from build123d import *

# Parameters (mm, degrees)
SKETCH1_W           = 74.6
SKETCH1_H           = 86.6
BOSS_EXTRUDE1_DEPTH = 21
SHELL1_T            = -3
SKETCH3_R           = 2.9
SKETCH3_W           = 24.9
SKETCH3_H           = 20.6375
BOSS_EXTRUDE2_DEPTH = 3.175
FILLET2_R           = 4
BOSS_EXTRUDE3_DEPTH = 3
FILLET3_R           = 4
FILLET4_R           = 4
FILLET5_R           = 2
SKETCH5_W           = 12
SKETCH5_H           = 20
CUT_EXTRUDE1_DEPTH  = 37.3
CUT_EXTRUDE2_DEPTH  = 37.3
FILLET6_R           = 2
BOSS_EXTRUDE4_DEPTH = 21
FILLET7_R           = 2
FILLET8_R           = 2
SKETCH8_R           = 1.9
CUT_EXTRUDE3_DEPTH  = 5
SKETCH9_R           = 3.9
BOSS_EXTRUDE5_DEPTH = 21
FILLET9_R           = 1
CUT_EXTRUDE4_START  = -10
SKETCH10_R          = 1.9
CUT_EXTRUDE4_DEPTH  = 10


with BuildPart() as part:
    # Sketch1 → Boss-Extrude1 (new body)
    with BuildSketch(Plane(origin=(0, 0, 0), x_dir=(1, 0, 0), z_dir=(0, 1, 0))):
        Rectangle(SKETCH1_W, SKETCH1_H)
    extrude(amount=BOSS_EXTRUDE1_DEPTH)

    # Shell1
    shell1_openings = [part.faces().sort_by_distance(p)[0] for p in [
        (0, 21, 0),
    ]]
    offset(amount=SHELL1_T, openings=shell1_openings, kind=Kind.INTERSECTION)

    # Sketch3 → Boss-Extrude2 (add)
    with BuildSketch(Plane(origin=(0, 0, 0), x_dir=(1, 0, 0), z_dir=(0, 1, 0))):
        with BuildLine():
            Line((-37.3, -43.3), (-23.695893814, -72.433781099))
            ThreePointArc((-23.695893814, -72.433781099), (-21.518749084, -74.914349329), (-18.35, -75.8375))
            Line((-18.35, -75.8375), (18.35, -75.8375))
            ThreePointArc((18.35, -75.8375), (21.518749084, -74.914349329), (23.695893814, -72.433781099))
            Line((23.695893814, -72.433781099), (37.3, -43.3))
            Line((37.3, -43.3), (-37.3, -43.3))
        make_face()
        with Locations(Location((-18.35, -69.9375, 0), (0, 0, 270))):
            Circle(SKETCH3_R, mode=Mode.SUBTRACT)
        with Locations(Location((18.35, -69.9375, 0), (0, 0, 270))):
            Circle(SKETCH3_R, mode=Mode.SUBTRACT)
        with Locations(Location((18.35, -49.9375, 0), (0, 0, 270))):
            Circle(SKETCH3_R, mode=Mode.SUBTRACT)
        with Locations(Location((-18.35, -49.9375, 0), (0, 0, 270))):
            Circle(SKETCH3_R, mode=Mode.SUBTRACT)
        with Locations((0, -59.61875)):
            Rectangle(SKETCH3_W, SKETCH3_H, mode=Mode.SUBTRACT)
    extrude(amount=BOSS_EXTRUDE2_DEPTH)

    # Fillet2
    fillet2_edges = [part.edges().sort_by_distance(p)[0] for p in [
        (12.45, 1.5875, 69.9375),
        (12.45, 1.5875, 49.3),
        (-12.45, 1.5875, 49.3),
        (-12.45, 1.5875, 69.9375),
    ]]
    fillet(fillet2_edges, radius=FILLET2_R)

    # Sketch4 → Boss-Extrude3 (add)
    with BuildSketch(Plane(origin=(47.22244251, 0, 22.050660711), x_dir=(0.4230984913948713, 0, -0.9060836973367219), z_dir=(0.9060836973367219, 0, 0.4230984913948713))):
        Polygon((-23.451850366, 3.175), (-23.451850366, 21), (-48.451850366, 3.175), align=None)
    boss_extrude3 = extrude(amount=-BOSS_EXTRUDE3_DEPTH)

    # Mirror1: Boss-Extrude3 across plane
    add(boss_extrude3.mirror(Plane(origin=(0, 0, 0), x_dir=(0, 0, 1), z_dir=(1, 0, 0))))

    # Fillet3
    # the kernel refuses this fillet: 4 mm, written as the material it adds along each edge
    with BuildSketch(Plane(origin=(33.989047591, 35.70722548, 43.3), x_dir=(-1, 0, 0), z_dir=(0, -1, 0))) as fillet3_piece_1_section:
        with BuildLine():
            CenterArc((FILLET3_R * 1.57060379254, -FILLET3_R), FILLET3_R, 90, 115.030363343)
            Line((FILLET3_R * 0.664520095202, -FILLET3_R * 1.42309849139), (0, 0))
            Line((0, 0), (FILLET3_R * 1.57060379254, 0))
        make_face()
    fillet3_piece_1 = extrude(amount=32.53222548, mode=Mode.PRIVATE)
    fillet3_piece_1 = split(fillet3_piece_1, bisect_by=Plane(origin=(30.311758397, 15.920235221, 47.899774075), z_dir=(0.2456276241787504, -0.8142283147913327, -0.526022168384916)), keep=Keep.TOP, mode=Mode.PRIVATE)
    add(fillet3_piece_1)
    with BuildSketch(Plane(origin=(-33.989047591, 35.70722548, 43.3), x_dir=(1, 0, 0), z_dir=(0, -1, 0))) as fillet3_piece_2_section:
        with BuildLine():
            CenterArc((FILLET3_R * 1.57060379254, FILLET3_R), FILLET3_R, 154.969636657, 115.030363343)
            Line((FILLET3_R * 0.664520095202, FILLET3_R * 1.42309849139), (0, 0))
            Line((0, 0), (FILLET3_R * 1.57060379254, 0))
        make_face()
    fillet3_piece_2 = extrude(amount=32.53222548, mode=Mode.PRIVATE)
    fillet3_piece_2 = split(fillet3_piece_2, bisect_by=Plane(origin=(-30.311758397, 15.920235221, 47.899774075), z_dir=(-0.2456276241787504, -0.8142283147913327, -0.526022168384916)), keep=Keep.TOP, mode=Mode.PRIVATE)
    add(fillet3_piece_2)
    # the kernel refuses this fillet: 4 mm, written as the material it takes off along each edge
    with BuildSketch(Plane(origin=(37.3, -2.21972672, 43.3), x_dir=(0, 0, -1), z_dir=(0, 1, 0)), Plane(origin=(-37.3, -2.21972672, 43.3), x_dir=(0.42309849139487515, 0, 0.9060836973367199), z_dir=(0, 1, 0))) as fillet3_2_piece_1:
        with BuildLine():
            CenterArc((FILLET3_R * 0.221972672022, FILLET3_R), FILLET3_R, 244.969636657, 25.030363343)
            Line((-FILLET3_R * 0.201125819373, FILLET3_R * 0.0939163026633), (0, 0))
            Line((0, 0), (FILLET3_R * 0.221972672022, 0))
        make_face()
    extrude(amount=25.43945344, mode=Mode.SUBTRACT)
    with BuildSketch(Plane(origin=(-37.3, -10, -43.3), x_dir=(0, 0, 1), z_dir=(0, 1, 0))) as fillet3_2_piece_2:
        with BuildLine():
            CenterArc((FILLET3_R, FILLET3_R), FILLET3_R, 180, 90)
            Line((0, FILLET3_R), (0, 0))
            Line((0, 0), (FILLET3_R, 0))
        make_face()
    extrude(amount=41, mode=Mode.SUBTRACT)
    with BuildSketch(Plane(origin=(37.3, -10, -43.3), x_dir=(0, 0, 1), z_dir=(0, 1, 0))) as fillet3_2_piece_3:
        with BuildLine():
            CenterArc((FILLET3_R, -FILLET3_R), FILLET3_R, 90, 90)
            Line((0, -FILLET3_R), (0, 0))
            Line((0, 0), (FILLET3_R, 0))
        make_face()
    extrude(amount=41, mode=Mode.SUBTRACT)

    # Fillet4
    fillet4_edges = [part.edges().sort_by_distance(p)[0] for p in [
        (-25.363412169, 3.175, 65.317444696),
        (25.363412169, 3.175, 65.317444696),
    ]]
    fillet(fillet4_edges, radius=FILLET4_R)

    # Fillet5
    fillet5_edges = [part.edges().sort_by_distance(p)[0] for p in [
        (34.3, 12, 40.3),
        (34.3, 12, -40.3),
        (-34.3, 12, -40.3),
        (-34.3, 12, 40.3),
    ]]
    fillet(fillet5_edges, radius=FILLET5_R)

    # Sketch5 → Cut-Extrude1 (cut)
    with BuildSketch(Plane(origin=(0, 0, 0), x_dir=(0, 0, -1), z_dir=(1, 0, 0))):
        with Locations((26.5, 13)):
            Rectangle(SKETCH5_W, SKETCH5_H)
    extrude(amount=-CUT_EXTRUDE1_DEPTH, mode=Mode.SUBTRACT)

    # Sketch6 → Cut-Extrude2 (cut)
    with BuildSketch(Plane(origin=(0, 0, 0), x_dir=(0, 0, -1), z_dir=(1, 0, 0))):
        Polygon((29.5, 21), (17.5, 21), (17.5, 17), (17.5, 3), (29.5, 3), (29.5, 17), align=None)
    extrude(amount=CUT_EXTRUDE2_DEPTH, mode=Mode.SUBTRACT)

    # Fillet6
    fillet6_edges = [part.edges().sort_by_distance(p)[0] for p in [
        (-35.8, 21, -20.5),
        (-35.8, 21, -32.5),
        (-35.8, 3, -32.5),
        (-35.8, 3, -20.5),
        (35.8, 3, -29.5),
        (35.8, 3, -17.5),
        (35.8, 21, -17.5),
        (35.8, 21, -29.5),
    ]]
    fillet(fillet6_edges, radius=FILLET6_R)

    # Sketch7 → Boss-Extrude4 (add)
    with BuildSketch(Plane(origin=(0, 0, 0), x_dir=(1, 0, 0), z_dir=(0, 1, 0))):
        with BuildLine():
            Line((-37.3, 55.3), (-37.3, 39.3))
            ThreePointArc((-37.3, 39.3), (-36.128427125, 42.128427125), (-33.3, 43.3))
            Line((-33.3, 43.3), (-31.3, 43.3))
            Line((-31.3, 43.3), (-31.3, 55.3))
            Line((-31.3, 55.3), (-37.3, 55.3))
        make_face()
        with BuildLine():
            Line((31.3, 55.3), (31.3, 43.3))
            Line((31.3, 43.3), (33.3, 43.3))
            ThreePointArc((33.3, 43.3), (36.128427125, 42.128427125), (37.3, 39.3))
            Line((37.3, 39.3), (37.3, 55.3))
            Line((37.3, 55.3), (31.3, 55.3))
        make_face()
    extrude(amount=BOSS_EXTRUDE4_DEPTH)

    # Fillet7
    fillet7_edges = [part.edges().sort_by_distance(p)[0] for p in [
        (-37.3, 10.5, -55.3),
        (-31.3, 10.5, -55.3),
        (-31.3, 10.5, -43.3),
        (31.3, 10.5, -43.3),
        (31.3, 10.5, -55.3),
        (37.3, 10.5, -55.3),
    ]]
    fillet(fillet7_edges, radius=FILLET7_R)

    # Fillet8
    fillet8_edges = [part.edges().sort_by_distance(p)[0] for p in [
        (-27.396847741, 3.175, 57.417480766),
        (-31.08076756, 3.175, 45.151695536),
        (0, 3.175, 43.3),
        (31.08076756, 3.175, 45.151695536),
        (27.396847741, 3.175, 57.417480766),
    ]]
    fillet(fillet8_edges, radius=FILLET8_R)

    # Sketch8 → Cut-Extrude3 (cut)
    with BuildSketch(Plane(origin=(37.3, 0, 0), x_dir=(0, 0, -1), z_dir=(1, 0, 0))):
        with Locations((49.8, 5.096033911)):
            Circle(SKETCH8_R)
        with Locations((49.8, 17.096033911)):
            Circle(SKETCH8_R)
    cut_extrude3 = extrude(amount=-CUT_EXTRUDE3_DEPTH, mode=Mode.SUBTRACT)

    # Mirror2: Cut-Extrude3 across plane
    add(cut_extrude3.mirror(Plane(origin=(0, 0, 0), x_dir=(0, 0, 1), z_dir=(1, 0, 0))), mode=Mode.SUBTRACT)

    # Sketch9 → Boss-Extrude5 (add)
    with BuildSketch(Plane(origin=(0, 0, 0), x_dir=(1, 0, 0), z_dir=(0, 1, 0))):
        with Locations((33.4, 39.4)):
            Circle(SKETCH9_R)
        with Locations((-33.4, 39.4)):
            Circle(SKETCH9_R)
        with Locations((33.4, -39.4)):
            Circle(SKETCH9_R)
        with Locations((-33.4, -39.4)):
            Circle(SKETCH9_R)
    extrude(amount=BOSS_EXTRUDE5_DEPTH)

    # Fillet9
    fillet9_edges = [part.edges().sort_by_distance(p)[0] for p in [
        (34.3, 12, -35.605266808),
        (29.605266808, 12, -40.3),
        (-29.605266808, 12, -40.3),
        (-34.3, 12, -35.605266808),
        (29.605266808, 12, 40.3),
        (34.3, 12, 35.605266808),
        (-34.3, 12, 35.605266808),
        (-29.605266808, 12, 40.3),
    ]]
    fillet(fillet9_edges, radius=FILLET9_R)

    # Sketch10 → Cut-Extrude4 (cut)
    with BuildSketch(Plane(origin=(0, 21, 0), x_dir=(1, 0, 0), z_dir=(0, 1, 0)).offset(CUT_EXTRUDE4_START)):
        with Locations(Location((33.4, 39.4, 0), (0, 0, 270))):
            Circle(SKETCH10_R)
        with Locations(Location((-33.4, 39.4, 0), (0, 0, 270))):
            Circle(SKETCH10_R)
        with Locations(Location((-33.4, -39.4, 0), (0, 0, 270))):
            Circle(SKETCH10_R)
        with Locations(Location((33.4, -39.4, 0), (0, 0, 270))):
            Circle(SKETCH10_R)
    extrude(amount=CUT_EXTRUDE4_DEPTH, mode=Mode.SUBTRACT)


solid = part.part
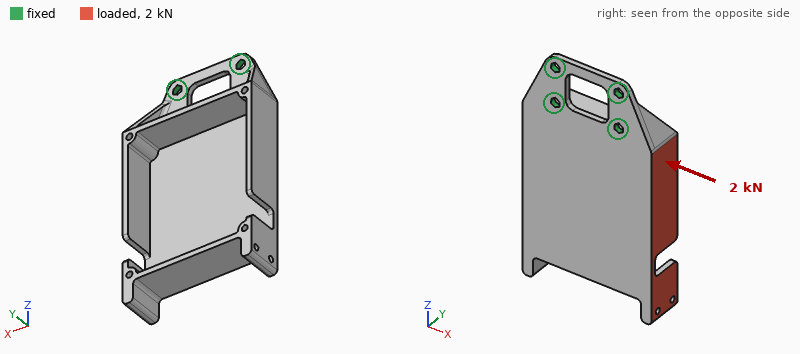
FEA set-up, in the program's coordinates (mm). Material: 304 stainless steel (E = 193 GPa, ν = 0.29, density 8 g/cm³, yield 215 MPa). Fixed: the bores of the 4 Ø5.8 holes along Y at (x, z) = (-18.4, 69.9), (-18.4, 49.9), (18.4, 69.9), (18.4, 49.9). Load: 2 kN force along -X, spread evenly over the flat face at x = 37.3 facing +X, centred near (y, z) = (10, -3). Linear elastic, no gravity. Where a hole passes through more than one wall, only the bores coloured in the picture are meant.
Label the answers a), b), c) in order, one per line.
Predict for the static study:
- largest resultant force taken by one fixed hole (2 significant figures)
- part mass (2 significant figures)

a) 2.5 kN
b) 360 g
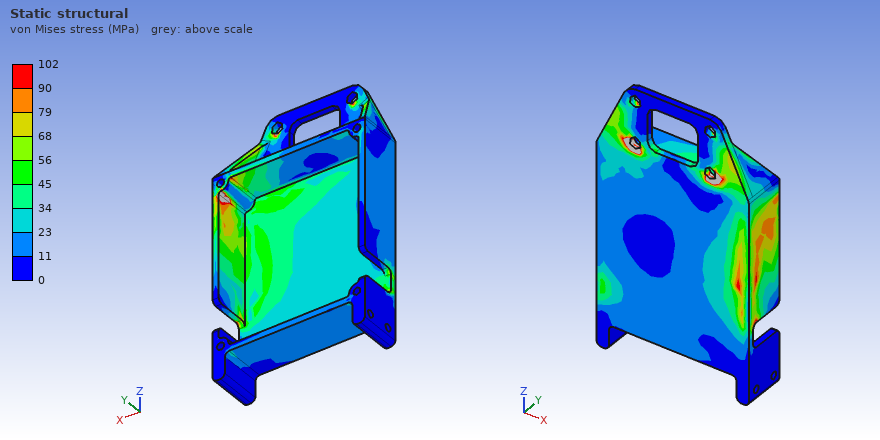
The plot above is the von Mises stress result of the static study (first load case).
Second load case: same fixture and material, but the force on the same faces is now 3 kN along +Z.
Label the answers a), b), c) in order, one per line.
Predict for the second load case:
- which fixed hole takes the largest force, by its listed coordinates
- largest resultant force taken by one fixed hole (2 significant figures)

a) (18.4, 49.9)
b) 2.7 kN
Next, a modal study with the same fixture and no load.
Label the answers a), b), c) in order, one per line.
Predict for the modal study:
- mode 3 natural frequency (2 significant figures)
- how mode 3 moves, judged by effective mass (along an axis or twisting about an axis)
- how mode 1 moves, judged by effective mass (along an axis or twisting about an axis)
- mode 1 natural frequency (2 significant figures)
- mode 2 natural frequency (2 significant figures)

a) 1500 Hz
b) along Y
c) along Y
d) 490 Hz
e) 780 Hz
